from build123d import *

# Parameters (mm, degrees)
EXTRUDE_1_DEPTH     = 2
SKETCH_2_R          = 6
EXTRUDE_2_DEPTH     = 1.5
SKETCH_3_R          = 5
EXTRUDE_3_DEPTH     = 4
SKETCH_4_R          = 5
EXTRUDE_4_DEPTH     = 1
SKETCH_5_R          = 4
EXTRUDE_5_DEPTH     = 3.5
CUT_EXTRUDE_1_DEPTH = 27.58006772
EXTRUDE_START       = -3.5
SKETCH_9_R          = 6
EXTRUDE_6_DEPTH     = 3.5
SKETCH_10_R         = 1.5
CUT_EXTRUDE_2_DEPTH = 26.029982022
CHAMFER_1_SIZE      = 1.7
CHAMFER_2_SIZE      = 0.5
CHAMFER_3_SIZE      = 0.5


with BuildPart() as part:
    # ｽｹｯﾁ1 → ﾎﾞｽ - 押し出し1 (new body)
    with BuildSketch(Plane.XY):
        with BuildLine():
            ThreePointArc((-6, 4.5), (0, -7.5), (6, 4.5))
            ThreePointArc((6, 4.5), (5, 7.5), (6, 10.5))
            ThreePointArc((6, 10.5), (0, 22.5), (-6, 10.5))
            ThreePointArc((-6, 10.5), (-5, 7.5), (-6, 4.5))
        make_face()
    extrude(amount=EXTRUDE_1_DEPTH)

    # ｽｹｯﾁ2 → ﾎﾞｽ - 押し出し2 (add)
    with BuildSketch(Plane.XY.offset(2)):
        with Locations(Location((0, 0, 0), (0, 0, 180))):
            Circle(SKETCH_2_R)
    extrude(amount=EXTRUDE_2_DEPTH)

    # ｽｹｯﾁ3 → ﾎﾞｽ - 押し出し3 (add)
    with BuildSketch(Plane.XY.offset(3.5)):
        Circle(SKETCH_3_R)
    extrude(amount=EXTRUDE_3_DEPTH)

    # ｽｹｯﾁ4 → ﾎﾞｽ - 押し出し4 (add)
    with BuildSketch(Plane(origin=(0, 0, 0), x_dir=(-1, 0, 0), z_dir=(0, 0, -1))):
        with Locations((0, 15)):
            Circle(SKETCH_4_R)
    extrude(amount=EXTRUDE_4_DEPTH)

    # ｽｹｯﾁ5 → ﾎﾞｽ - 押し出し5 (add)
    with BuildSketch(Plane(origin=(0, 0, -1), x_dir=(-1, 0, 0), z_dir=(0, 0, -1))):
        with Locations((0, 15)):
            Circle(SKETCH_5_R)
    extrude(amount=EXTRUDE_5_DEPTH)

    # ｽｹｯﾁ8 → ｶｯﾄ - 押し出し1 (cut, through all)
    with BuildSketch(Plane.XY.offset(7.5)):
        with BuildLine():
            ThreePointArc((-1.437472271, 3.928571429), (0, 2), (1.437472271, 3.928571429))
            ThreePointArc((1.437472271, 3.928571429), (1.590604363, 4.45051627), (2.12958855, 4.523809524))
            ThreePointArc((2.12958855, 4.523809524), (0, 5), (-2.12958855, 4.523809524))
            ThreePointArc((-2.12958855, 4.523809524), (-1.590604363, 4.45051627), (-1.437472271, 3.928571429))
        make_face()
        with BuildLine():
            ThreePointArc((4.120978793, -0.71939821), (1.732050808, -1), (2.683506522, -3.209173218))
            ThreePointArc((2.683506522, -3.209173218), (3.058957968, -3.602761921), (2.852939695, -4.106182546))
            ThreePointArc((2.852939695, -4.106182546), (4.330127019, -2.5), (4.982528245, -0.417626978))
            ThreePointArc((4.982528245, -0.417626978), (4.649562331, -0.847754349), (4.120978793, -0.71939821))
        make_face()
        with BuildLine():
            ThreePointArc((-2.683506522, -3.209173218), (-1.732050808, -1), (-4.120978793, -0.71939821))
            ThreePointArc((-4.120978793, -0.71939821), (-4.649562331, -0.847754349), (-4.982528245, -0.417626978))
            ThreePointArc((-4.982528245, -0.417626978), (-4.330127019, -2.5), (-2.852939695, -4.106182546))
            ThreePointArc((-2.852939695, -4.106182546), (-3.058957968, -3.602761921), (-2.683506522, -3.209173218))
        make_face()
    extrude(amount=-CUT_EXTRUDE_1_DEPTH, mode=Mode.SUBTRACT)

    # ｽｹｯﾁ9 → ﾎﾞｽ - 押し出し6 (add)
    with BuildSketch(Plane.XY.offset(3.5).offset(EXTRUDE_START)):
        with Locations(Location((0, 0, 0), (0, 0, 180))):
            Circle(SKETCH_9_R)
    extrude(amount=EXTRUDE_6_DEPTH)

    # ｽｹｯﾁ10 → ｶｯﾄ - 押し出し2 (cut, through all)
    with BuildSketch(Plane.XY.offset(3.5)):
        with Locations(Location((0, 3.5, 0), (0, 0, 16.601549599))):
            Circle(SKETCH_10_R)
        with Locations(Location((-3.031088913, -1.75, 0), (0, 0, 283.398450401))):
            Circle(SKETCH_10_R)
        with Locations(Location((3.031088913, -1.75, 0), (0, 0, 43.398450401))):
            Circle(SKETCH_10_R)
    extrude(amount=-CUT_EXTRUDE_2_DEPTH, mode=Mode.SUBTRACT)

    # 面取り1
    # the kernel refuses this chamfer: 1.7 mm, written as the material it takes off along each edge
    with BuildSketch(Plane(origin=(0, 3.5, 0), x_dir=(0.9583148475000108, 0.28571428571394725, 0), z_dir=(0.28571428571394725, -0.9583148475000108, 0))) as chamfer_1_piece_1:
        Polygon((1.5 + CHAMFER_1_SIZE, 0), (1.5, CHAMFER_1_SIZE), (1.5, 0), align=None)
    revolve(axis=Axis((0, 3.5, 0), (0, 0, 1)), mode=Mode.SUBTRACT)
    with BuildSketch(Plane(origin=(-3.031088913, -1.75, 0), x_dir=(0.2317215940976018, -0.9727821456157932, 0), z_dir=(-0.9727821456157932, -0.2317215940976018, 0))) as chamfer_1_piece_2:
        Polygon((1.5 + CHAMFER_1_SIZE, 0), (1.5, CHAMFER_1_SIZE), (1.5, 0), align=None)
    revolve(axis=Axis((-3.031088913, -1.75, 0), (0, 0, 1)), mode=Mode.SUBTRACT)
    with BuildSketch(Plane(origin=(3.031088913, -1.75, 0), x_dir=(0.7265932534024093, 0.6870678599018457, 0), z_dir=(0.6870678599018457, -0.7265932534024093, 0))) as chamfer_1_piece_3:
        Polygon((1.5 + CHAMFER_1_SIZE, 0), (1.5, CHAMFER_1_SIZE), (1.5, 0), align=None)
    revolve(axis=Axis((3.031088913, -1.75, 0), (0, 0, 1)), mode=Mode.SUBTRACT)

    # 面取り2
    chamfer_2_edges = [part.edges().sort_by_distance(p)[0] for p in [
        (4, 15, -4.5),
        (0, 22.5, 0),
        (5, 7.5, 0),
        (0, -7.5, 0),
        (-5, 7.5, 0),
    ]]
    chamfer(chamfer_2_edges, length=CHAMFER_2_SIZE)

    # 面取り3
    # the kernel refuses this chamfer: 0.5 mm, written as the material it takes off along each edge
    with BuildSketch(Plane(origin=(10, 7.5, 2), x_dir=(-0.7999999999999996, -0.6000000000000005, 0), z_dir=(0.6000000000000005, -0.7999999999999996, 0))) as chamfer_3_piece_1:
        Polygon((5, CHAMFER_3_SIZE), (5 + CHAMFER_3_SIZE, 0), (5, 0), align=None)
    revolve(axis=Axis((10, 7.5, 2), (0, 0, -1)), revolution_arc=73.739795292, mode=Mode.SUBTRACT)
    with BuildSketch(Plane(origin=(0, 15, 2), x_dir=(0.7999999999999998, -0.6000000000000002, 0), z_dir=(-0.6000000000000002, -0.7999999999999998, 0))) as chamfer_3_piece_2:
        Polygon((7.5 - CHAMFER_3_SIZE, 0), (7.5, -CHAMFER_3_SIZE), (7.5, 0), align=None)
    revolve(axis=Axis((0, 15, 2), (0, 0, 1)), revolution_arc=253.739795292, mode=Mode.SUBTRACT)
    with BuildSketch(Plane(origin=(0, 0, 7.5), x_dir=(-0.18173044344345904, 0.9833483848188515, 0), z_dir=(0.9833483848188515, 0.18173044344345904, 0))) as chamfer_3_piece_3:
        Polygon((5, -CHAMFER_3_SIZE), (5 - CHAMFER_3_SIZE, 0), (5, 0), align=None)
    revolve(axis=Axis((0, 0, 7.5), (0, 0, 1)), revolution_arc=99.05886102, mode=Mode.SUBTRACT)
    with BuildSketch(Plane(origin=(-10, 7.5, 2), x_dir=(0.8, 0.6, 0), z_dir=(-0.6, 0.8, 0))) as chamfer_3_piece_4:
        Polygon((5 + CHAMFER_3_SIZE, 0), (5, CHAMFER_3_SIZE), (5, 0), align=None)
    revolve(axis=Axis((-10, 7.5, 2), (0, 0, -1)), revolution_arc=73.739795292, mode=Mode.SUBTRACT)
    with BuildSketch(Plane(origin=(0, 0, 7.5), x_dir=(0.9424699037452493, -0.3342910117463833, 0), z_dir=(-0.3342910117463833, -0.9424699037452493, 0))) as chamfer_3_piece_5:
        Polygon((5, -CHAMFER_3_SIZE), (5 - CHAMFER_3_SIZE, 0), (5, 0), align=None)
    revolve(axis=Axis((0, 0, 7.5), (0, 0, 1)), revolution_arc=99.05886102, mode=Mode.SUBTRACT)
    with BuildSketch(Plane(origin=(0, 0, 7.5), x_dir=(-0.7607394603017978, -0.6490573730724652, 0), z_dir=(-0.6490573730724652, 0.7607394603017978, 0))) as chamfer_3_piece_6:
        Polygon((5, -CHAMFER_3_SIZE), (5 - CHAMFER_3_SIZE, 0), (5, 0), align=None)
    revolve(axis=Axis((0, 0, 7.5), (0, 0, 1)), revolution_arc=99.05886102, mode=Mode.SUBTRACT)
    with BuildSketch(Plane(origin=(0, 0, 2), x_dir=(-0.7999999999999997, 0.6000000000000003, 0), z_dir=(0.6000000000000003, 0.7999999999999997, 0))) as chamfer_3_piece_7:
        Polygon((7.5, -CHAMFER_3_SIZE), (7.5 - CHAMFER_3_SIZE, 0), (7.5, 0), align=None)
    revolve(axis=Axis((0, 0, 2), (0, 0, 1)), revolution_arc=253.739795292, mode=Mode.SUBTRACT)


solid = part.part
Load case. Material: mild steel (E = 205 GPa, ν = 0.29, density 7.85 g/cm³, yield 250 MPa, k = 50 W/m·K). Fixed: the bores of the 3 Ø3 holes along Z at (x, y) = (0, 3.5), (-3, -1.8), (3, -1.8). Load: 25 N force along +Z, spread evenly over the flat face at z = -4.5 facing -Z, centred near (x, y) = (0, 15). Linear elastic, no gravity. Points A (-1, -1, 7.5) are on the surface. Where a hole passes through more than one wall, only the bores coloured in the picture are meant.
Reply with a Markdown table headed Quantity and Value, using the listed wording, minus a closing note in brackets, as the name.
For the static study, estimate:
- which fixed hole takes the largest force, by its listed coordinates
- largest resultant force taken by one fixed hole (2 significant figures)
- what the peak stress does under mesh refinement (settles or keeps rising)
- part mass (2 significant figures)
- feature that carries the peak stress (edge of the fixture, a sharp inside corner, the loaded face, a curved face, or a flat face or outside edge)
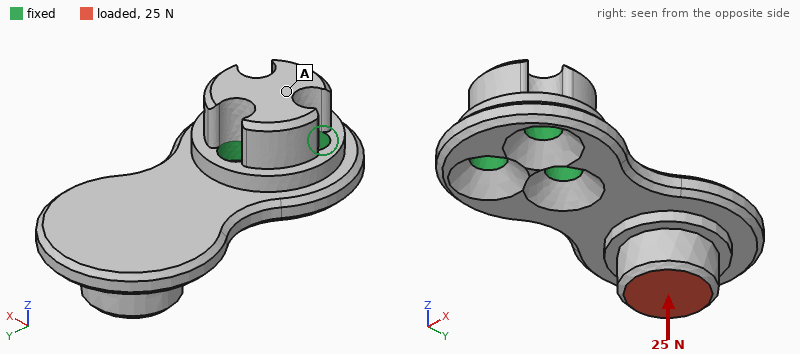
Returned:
| Quantity | Value |
|---|---|
| which fixed hole takes the largest force, by its listed coordinates | (0, 3.5) |
| largest resultant force taken by one fixed hole | 77 N |
| what the peak stress does under mesh refinement | keeps rising |
| part mass | 9.6 g |
| feature that carries the peak stress | a sharp inside corner |
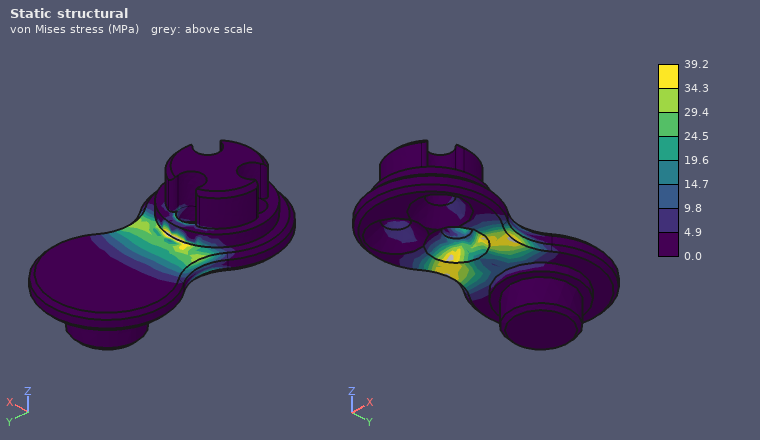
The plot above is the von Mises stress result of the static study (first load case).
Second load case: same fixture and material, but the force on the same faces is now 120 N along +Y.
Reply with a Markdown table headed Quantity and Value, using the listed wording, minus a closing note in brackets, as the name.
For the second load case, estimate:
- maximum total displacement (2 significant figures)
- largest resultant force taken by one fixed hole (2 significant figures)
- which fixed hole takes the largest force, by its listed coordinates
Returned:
| Quantity | Value |
|---|---|
| maximum total displacement | 59 µm |
| largest resultant force taken by one fixed hole | 130 N |
| which fixed hole takes the largest force, by its listed coordinates | (0, 3.5) |
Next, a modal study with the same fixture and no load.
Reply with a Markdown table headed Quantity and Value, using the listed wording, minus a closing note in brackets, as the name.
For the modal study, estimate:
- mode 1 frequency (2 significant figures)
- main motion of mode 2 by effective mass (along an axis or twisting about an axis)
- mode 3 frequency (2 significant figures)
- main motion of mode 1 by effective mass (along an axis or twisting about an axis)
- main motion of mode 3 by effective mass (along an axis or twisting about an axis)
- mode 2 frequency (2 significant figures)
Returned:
| Quantity | Value |
|---|---|
| mode 1 frequency | 3600 Hz |
| main motion of mode 2 by effective mass | along X |
| mode 3 frequency | 15 kHz |
| main motion of mode 1 by effective mass | along Z |
| main motion of mode 3 by effective mass | along X |
| mode 2 frequency | 11 kHz |
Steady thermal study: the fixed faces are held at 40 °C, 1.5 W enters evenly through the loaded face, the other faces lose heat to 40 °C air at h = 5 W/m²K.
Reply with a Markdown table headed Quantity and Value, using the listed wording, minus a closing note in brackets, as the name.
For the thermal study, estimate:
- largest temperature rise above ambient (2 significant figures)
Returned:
| Quantity | Value |
|---|---|
| largest temperature rise above ambient | 16 K |
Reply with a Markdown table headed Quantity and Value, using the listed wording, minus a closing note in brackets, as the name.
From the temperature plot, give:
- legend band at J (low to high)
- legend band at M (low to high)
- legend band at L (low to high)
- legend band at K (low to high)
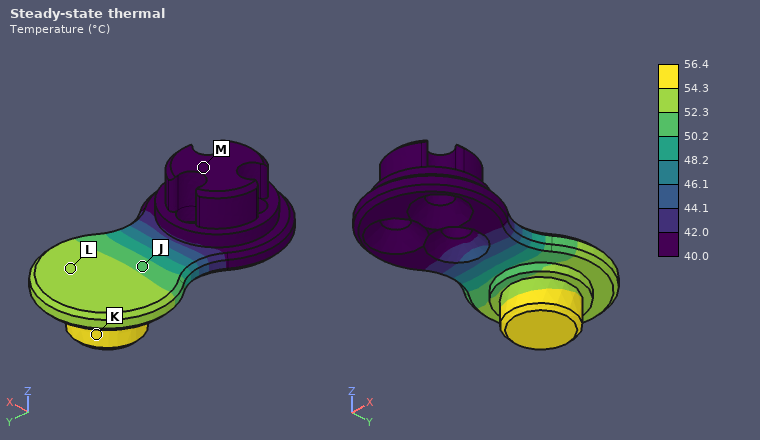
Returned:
| Quantity | Value |
|---|---|
| legend band at J | 50.2 to 52.3 °C |
| legend band at M | 40.0 to 42.0 °C |
| legend band at L | 52.3 to 54.3 °C |
| legend band at K | 54.3 to 56.4 °C |
